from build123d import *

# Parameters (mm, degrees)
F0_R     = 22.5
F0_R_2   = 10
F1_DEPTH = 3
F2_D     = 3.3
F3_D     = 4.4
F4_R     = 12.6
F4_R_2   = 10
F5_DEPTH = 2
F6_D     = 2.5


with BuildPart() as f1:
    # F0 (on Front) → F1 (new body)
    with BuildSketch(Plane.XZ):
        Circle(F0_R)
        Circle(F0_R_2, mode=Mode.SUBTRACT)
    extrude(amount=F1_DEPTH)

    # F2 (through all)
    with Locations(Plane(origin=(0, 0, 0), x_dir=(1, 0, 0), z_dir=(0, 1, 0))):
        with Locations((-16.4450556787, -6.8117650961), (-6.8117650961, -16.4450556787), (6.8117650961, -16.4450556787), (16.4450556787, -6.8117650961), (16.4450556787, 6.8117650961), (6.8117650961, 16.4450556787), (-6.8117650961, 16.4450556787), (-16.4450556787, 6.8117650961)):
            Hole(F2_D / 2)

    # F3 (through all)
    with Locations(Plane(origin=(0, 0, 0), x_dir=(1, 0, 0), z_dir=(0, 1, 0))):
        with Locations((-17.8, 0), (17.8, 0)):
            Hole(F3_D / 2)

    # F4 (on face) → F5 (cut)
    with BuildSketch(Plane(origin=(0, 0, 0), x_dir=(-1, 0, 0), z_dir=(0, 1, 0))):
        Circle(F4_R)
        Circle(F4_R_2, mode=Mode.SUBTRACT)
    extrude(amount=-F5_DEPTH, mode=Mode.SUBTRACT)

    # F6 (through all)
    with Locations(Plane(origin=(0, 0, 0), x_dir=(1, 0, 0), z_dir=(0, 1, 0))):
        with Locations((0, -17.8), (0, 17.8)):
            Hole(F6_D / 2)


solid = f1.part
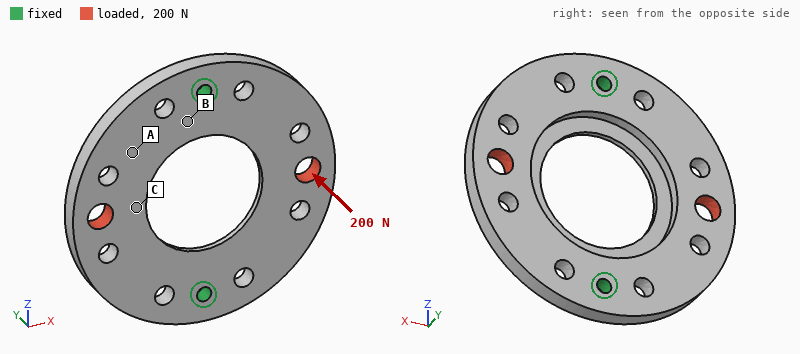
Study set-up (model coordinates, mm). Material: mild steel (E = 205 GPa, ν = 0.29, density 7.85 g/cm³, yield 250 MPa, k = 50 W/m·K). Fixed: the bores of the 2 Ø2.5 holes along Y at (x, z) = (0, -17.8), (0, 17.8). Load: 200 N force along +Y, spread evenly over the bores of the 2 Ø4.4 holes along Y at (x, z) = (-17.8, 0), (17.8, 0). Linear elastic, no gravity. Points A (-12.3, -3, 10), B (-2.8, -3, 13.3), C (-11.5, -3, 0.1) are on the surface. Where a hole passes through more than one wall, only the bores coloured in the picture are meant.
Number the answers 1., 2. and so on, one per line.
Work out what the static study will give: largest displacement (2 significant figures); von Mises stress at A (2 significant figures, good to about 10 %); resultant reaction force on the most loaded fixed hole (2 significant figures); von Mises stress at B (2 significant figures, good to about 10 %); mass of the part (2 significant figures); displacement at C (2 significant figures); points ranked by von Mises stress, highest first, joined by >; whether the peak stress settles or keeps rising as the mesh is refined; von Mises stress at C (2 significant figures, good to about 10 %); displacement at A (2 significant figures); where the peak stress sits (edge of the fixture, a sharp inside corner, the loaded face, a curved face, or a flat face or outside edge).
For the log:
1. 40 µm
2. 17 MPa
3. 120 N
4. 50 MPa
5. 25 g
6. 18 µm
7. B > C > A
8. keeps rising
9. 30 MPa
10. 15 µm
11. edge of the fixture
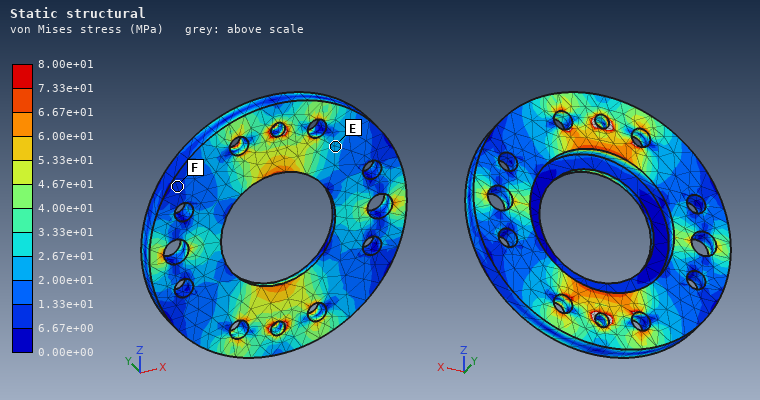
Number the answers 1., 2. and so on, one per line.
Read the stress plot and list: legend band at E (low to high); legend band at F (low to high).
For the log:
1. 2.00e+01 to 2.67e+01 MPa
2. 6.67e+00 to 1.33e+01 MPa
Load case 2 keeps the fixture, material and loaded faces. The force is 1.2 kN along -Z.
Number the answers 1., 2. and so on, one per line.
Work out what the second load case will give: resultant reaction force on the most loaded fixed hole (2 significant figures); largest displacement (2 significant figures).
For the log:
1. 600 N
2. 4.4 µm
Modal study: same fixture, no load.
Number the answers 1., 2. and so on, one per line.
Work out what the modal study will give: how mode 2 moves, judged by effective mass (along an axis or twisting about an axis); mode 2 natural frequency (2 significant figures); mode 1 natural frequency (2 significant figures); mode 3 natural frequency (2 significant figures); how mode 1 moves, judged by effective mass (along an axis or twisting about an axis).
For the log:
1. along Y
2. 4400 Hz
3. 3900 Hz
4. 10 kHz
5. twisting about Z
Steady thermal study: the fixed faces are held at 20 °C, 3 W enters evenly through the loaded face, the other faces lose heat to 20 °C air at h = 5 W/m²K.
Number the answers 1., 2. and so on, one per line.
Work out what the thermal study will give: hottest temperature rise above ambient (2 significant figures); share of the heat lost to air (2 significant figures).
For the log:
1. 15 K
2. 3.9 %
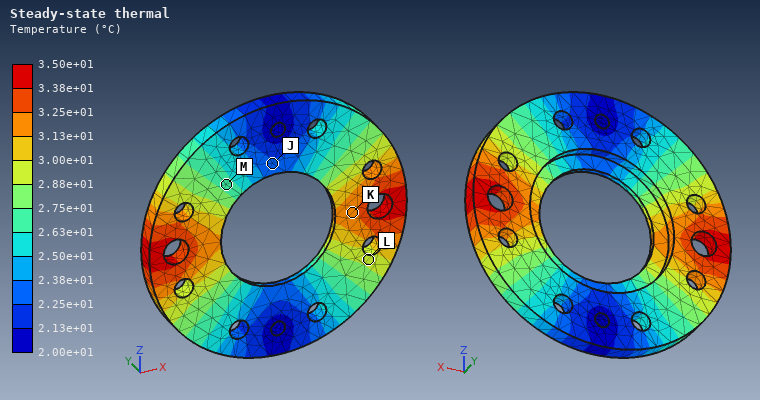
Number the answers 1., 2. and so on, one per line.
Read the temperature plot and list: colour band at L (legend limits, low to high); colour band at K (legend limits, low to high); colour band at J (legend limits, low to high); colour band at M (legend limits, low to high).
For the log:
1. 2.88e+01 to 3.00e+01 °C
2. 3.13e+01 to 3.25e+01 °C
3. 2.25e+01 to 2.38e+01 °C
4. 2.63e+01 to 2.75e+01 °C
